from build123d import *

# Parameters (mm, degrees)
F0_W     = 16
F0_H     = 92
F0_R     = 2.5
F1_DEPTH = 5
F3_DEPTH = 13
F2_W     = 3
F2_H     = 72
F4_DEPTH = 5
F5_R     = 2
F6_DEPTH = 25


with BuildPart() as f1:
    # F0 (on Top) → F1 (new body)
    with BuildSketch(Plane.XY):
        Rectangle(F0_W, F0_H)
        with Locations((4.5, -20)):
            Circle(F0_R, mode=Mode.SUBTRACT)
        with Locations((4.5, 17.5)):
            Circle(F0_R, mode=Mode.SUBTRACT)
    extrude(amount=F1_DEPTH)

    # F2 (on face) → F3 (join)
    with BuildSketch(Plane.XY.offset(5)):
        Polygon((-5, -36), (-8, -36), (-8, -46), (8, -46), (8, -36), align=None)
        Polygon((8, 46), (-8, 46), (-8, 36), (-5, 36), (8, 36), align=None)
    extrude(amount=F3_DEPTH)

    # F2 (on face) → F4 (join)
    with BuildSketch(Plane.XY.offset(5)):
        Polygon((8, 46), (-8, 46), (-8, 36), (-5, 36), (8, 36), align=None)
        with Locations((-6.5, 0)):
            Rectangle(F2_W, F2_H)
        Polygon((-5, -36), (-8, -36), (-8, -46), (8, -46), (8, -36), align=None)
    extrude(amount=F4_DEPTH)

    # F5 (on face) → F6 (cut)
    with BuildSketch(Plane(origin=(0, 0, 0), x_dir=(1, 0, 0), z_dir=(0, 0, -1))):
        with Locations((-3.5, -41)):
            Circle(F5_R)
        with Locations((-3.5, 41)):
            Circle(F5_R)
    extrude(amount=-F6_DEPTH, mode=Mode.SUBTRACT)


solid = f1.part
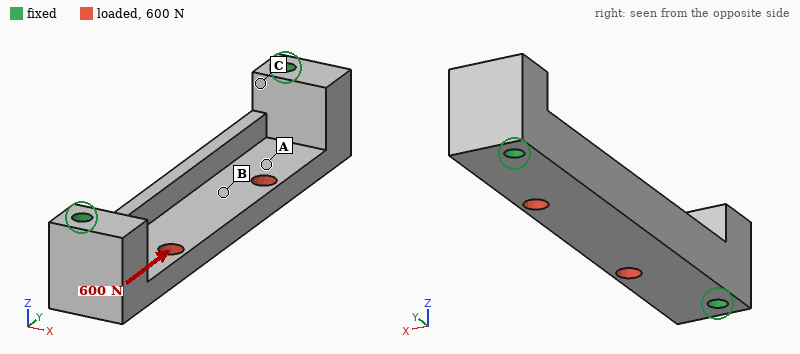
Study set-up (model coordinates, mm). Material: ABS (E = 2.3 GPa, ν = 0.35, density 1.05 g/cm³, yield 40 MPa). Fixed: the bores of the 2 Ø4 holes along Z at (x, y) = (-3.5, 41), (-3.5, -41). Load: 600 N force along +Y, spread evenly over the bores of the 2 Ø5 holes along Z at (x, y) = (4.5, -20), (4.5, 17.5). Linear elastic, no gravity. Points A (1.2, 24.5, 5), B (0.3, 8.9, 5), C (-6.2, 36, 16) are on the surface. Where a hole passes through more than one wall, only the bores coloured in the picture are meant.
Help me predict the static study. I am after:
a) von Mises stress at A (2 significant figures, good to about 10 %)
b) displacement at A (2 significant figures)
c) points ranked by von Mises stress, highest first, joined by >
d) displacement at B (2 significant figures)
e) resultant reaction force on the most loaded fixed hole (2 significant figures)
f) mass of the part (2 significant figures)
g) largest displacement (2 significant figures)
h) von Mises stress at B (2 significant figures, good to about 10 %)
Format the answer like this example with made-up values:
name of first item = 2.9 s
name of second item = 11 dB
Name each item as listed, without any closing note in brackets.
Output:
von Mises stress at A = 3.7 MPa
displacement at A = 28 µm
points ranked by von Mises stress, highest first, joined by > = A > B > C
displacement at B = 39 µm
resultant reaction force on the most loaded fixed hole = 310 N
mass of the part = 13 g
largest displacement = 56 µm
von Mises stress at B = 2.0 MPa
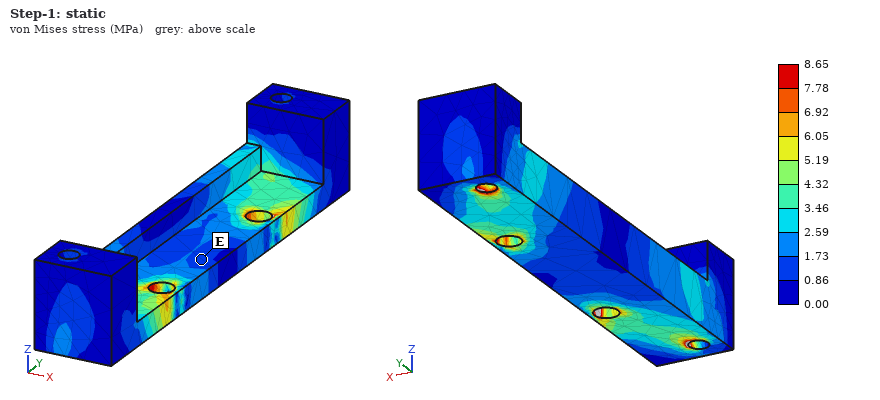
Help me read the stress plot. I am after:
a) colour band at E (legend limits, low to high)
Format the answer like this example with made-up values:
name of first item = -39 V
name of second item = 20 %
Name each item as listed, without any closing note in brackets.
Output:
colour band at E = 0.86 to 1.73 MPa
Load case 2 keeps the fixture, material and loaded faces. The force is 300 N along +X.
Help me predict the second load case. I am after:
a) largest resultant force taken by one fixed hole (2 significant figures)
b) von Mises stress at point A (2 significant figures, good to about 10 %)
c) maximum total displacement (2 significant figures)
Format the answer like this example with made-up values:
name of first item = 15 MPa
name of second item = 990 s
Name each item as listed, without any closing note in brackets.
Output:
largest resultant force taken by one fixed hole = 160 N
von Mises stress at point A = 4.4 MPa
maximum total displacement = 0.26 mm
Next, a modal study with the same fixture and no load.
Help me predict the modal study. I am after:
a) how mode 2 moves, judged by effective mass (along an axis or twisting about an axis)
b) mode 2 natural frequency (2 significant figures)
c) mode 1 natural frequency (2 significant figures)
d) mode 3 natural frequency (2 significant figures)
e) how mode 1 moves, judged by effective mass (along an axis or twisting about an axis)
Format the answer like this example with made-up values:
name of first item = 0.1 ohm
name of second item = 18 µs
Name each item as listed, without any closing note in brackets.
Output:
how mode 2 moves, judged by effective mass = along X
mode 2 natural frequency = 2400 Hz
mode 1 natural frequency = 1700 Hz
mode 3 natural frequency = 3400 Hz
how mode 1 moves, judged by effective mass = along Z
